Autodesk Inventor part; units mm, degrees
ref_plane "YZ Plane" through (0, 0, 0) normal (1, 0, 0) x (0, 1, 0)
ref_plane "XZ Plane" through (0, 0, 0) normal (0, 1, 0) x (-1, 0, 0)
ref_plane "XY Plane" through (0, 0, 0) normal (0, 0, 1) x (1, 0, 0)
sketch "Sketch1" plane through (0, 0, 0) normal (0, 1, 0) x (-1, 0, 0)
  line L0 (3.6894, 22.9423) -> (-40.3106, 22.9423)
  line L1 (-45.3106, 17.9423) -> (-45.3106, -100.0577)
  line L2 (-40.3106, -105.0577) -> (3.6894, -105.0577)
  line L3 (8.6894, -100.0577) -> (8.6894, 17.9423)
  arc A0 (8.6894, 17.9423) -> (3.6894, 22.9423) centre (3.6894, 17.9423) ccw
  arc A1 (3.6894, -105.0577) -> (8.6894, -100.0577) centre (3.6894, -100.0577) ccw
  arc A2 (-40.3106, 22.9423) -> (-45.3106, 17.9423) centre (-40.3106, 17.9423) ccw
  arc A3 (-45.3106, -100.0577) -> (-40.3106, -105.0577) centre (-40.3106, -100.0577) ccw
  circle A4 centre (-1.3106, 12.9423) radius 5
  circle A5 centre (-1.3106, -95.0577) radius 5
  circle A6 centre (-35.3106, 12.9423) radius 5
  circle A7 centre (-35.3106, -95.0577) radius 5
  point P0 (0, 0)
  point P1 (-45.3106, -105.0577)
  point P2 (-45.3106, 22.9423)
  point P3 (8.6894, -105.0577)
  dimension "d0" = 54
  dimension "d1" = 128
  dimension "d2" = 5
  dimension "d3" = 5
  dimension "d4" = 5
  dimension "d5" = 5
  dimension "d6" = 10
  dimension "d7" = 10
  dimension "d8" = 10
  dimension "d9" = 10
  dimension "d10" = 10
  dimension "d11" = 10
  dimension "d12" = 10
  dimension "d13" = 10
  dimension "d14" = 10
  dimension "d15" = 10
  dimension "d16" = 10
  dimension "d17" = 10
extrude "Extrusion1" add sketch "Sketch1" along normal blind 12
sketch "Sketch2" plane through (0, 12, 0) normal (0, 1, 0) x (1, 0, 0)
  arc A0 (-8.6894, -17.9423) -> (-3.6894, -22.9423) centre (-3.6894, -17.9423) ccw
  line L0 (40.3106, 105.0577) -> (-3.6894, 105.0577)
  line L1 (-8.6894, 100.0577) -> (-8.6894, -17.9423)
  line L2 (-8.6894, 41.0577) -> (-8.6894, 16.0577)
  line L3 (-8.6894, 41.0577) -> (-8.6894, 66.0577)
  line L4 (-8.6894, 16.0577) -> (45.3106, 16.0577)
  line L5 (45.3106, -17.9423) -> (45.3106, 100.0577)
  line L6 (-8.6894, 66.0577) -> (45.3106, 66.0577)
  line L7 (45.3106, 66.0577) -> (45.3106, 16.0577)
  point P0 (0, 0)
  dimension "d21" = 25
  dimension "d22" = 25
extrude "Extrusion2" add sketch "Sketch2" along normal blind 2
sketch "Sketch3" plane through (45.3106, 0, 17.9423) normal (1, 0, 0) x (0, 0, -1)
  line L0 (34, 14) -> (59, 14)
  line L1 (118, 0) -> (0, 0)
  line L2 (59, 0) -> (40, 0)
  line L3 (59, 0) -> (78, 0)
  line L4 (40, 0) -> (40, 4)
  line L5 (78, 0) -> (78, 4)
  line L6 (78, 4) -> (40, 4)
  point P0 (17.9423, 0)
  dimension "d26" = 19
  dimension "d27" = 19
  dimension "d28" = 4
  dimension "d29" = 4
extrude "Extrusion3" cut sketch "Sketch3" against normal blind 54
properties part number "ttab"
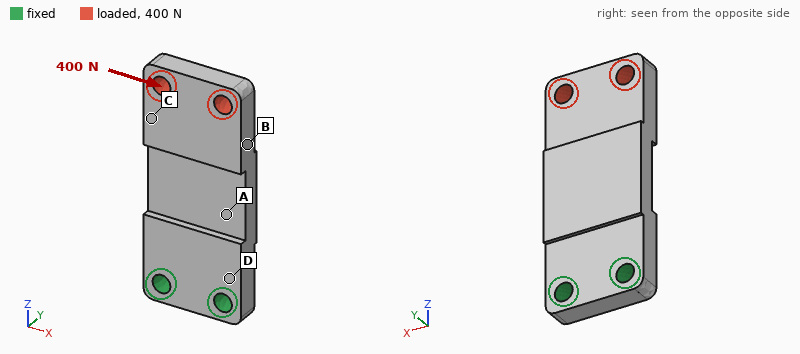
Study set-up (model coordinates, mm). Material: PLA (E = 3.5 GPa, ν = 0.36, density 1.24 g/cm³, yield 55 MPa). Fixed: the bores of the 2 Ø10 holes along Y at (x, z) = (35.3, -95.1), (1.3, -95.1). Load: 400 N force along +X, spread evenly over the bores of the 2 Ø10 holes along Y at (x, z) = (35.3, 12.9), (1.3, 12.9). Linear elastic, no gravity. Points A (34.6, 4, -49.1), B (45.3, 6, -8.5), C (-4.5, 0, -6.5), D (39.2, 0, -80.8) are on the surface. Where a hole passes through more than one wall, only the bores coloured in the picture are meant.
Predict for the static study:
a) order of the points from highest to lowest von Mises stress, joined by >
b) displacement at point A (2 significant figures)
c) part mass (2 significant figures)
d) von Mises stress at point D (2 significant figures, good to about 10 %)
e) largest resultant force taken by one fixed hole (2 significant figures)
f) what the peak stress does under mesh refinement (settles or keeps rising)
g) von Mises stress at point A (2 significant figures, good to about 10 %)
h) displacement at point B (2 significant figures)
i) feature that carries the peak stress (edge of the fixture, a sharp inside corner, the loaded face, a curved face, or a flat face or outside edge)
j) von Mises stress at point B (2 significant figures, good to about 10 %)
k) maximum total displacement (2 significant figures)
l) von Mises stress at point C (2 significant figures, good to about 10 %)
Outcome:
A > D > B > C
0.12 mm
94 g
3.8 MPa
1.1 kN
keeps rising
4.8 MPa
0.34 mm
edge of the fixture
1.5 MPa
0.50 mm
0.82 MPa
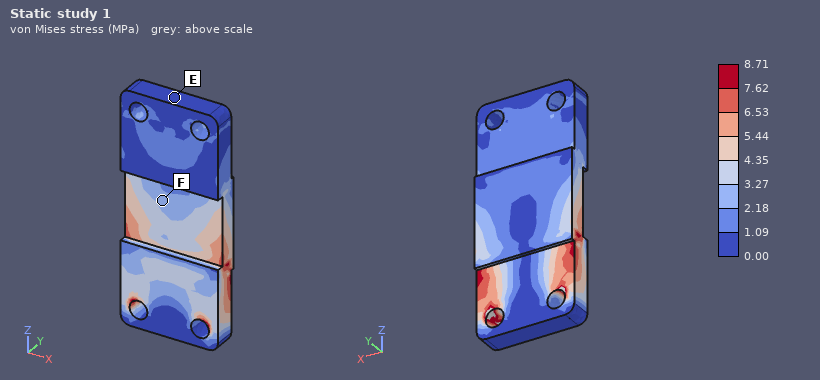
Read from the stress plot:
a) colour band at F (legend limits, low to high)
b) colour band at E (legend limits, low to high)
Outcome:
2.18 to 3.27 MPa
0.00 to 1.09 MPa
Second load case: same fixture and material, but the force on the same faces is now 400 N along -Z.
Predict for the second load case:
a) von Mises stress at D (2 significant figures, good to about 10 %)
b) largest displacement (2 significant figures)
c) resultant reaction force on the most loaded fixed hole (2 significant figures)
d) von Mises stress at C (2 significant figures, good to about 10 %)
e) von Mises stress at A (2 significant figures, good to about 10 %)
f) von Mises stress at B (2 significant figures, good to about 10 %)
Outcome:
0.69 MPa
0.21 mm
200 N
0.70 MPa
2.0 MPa
0.77 MPa
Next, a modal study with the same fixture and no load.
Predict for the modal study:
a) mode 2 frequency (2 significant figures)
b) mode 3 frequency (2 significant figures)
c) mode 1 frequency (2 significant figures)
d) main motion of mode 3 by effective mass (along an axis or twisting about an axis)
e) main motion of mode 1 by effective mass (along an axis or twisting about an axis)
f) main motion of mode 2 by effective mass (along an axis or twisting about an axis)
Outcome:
850 Hz
1000 Hz
230 Hz
along X
along Y
along X
